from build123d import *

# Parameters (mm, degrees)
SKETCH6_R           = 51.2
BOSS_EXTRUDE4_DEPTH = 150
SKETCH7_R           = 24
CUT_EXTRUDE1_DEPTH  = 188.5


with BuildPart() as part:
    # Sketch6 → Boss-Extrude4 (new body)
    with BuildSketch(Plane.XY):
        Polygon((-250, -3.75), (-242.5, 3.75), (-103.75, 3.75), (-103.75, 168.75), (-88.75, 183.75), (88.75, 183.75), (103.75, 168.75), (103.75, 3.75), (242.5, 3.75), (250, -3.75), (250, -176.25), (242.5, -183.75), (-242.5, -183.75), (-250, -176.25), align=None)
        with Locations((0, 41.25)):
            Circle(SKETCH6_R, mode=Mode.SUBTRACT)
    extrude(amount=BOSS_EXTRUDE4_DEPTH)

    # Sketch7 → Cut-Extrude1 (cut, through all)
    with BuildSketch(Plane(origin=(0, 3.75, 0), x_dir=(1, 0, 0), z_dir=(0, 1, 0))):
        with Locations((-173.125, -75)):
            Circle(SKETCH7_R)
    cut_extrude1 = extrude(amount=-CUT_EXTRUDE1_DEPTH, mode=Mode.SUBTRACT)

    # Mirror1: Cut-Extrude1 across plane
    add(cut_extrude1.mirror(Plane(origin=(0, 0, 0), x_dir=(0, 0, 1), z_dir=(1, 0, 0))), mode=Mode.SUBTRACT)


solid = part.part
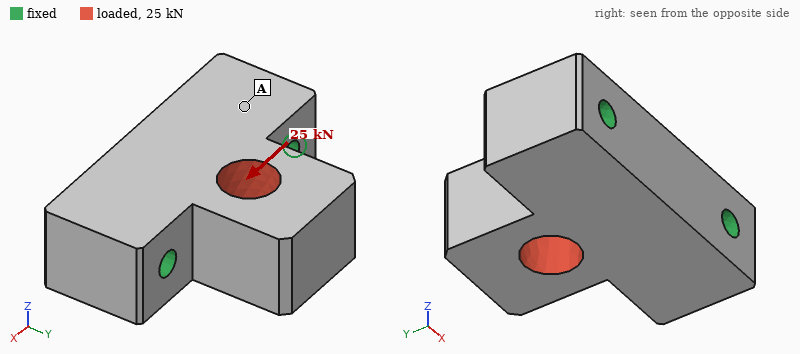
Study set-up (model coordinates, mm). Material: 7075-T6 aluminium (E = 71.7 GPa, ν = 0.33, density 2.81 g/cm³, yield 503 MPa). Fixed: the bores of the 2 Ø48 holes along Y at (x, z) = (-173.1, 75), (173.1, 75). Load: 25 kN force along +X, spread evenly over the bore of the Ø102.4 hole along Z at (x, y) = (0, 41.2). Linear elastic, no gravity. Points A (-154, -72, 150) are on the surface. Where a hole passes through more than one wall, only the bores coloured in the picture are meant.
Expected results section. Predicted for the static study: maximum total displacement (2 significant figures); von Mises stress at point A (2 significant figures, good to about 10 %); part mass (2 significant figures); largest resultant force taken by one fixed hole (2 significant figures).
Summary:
9.4 µm
0.59 MPa
50 kg
15 kN
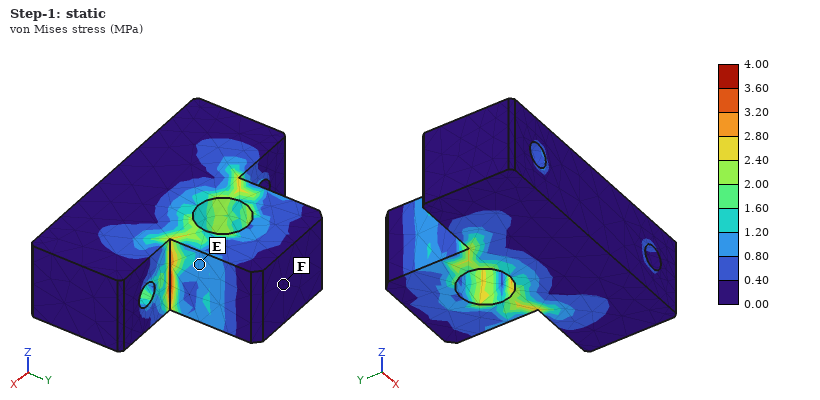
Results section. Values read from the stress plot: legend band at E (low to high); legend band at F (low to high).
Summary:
0.80 to 1.20 MPa
0.00 to 0.40 MPa
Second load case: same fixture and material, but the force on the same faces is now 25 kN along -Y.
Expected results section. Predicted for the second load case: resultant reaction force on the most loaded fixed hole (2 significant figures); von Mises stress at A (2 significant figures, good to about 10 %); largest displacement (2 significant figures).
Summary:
13 kN
0.55 MPa
3.9 µm
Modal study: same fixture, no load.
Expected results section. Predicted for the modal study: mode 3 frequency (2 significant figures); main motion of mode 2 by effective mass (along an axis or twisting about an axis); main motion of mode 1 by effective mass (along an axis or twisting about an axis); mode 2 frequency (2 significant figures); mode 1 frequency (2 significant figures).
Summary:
2500 Hz
along X
along Z
1800 Hz
1100 Hz
